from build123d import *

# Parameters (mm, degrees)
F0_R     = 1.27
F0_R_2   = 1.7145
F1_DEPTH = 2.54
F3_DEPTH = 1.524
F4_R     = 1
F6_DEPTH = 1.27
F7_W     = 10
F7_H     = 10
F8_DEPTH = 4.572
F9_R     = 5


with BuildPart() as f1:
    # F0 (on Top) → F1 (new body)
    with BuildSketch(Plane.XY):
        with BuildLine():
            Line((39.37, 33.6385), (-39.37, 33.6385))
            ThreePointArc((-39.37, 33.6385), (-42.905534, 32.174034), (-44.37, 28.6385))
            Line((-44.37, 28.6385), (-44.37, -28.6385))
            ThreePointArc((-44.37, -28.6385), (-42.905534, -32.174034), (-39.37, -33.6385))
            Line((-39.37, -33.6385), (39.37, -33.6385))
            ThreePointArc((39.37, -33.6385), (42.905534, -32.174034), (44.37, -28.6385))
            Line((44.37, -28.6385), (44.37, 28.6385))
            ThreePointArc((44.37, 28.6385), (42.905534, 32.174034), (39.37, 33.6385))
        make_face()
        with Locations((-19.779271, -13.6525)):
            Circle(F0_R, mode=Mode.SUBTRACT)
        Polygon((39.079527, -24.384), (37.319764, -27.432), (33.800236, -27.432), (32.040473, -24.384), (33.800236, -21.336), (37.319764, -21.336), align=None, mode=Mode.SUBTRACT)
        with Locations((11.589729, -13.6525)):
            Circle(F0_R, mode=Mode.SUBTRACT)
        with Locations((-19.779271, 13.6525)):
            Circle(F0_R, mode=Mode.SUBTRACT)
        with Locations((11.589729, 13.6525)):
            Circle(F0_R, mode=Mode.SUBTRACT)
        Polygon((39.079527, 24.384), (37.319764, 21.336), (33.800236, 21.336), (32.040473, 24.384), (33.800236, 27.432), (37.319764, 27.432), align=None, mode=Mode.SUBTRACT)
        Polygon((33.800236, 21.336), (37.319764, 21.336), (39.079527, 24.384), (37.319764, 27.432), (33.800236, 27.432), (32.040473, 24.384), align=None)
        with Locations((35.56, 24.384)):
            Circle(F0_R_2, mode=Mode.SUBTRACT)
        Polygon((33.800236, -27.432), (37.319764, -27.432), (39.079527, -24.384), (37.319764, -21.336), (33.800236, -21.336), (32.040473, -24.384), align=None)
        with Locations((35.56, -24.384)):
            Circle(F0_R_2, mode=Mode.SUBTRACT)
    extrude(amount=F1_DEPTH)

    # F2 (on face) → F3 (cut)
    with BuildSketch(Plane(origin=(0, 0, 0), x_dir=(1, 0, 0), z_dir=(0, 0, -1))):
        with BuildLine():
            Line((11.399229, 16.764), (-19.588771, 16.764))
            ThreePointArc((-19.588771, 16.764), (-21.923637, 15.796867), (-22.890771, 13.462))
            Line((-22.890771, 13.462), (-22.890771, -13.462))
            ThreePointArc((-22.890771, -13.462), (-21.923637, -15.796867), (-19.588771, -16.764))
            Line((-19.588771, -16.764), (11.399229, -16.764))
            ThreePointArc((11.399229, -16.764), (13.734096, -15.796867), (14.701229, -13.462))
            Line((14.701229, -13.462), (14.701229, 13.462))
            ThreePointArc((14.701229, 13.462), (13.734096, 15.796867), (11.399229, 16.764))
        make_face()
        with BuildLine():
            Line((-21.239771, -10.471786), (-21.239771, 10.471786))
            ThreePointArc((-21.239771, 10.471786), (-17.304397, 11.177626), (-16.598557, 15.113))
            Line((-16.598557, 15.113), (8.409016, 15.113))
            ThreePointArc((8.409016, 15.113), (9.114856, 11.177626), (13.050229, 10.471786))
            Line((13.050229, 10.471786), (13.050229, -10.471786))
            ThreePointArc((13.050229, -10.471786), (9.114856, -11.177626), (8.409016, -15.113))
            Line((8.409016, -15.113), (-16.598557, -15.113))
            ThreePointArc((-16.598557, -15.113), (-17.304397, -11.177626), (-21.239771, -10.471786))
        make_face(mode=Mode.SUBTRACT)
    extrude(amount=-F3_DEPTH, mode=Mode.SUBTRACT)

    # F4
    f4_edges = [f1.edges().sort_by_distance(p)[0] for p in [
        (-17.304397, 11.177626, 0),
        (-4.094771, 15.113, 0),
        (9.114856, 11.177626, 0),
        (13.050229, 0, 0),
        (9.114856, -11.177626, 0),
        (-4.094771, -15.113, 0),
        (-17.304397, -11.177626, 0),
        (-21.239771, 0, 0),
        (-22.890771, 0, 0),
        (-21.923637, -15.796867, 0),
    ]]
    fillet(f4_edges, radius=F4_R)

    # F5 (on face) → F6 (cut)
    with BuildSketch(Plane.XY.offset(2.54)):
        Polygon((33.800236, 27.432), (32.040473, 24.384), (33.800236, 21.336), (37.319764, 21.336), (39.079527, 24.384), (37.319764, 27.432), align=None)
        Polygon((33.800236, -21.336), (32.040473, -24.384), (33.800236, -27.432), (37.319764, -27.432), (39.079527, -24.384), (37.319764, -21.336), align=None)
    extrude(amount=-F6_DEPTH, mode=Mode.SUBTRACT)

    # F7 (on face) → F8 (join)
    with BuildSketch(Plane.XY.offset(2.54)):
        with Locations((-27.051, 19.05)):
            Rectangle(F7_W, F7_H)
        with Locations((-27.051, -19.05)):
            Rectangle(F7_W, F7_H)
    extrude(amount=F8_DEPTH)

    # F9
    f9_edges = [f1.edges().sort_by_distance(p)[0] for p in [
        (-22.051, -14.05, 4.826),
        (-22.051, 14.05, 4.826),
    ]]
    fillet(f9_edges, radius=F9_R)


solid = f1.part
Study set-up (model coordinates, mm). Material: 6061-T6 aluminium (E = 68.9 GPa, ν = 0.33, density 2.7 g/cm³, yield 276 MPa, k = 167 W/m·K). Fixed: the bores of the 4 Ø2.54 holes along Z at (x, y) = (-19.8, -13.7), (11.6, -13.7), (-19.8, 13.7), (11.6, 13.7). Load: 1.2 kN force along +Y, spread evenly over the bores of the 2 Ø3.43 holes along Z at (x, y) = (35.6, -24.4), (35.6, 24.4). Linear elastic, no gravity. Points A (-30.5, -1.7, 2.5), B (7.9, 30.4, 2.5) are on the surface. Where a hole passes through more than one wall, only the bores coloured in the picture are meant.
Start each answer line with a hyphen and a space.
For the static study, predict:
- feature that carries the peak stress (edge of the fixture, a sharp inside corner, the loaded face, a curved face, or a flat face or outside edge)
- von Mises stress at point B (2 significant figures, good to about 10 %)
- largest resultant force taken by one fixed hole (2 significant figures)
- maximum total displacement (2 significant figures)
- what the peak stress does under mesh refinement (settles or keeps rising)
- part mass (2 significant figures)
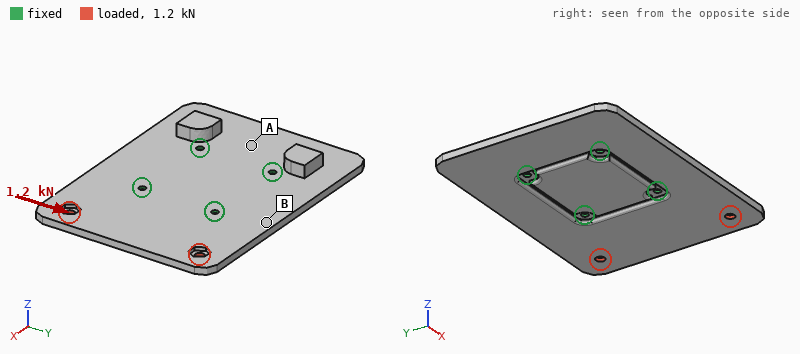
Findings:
- edge of the fixture
- 15 MPa
- 860 N
- 81 µm
- keeps rising
- 41 g
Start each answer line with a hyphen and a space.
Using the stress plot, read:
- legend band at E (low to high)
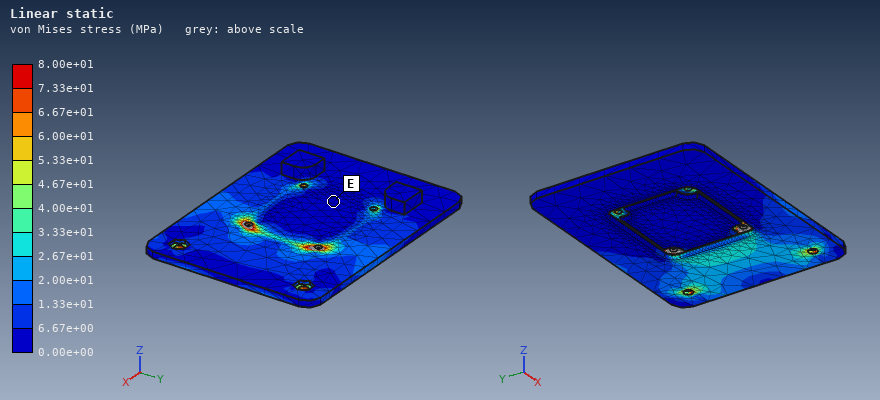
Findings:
- 0.00e+00 to 6.67e+00 MPa
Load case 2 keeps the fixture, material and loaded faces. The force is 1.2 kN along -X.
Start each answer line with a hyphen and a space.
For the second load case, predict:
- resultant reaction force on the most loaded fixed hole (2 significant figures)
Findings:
- 330 N
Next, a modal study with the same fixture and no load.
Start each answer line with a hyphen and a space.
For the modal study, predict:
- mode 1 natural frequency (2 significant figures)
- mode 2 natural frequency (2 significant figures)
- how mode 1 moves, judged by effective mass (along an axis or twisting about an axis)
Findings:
- 1200 Hz
- 2000 Hz
- along Z
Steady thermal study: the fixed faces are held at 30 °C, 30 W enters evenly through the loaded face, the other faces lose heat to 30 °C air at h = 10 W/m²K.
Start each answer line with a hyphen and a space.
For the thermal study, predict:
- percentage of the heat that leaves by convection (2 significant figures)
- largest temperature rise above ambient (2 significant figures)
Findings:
- 6.6 %
- 55 K
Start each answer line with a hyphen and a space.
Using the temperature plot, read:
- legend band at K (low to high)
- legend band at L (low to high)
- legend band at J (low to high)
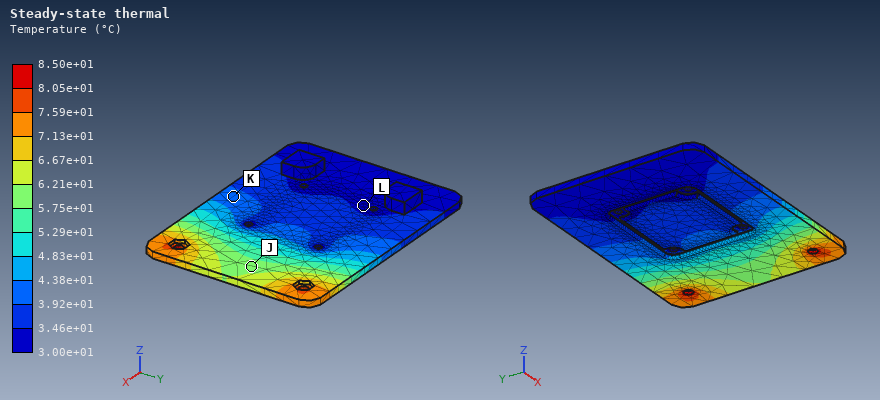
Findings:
- 3.92e+01 to 4.38e+01 °C
- 3.00e+01 to 3.46e+01 °C
- 5.75e+01 to 6.21e+01 °C
